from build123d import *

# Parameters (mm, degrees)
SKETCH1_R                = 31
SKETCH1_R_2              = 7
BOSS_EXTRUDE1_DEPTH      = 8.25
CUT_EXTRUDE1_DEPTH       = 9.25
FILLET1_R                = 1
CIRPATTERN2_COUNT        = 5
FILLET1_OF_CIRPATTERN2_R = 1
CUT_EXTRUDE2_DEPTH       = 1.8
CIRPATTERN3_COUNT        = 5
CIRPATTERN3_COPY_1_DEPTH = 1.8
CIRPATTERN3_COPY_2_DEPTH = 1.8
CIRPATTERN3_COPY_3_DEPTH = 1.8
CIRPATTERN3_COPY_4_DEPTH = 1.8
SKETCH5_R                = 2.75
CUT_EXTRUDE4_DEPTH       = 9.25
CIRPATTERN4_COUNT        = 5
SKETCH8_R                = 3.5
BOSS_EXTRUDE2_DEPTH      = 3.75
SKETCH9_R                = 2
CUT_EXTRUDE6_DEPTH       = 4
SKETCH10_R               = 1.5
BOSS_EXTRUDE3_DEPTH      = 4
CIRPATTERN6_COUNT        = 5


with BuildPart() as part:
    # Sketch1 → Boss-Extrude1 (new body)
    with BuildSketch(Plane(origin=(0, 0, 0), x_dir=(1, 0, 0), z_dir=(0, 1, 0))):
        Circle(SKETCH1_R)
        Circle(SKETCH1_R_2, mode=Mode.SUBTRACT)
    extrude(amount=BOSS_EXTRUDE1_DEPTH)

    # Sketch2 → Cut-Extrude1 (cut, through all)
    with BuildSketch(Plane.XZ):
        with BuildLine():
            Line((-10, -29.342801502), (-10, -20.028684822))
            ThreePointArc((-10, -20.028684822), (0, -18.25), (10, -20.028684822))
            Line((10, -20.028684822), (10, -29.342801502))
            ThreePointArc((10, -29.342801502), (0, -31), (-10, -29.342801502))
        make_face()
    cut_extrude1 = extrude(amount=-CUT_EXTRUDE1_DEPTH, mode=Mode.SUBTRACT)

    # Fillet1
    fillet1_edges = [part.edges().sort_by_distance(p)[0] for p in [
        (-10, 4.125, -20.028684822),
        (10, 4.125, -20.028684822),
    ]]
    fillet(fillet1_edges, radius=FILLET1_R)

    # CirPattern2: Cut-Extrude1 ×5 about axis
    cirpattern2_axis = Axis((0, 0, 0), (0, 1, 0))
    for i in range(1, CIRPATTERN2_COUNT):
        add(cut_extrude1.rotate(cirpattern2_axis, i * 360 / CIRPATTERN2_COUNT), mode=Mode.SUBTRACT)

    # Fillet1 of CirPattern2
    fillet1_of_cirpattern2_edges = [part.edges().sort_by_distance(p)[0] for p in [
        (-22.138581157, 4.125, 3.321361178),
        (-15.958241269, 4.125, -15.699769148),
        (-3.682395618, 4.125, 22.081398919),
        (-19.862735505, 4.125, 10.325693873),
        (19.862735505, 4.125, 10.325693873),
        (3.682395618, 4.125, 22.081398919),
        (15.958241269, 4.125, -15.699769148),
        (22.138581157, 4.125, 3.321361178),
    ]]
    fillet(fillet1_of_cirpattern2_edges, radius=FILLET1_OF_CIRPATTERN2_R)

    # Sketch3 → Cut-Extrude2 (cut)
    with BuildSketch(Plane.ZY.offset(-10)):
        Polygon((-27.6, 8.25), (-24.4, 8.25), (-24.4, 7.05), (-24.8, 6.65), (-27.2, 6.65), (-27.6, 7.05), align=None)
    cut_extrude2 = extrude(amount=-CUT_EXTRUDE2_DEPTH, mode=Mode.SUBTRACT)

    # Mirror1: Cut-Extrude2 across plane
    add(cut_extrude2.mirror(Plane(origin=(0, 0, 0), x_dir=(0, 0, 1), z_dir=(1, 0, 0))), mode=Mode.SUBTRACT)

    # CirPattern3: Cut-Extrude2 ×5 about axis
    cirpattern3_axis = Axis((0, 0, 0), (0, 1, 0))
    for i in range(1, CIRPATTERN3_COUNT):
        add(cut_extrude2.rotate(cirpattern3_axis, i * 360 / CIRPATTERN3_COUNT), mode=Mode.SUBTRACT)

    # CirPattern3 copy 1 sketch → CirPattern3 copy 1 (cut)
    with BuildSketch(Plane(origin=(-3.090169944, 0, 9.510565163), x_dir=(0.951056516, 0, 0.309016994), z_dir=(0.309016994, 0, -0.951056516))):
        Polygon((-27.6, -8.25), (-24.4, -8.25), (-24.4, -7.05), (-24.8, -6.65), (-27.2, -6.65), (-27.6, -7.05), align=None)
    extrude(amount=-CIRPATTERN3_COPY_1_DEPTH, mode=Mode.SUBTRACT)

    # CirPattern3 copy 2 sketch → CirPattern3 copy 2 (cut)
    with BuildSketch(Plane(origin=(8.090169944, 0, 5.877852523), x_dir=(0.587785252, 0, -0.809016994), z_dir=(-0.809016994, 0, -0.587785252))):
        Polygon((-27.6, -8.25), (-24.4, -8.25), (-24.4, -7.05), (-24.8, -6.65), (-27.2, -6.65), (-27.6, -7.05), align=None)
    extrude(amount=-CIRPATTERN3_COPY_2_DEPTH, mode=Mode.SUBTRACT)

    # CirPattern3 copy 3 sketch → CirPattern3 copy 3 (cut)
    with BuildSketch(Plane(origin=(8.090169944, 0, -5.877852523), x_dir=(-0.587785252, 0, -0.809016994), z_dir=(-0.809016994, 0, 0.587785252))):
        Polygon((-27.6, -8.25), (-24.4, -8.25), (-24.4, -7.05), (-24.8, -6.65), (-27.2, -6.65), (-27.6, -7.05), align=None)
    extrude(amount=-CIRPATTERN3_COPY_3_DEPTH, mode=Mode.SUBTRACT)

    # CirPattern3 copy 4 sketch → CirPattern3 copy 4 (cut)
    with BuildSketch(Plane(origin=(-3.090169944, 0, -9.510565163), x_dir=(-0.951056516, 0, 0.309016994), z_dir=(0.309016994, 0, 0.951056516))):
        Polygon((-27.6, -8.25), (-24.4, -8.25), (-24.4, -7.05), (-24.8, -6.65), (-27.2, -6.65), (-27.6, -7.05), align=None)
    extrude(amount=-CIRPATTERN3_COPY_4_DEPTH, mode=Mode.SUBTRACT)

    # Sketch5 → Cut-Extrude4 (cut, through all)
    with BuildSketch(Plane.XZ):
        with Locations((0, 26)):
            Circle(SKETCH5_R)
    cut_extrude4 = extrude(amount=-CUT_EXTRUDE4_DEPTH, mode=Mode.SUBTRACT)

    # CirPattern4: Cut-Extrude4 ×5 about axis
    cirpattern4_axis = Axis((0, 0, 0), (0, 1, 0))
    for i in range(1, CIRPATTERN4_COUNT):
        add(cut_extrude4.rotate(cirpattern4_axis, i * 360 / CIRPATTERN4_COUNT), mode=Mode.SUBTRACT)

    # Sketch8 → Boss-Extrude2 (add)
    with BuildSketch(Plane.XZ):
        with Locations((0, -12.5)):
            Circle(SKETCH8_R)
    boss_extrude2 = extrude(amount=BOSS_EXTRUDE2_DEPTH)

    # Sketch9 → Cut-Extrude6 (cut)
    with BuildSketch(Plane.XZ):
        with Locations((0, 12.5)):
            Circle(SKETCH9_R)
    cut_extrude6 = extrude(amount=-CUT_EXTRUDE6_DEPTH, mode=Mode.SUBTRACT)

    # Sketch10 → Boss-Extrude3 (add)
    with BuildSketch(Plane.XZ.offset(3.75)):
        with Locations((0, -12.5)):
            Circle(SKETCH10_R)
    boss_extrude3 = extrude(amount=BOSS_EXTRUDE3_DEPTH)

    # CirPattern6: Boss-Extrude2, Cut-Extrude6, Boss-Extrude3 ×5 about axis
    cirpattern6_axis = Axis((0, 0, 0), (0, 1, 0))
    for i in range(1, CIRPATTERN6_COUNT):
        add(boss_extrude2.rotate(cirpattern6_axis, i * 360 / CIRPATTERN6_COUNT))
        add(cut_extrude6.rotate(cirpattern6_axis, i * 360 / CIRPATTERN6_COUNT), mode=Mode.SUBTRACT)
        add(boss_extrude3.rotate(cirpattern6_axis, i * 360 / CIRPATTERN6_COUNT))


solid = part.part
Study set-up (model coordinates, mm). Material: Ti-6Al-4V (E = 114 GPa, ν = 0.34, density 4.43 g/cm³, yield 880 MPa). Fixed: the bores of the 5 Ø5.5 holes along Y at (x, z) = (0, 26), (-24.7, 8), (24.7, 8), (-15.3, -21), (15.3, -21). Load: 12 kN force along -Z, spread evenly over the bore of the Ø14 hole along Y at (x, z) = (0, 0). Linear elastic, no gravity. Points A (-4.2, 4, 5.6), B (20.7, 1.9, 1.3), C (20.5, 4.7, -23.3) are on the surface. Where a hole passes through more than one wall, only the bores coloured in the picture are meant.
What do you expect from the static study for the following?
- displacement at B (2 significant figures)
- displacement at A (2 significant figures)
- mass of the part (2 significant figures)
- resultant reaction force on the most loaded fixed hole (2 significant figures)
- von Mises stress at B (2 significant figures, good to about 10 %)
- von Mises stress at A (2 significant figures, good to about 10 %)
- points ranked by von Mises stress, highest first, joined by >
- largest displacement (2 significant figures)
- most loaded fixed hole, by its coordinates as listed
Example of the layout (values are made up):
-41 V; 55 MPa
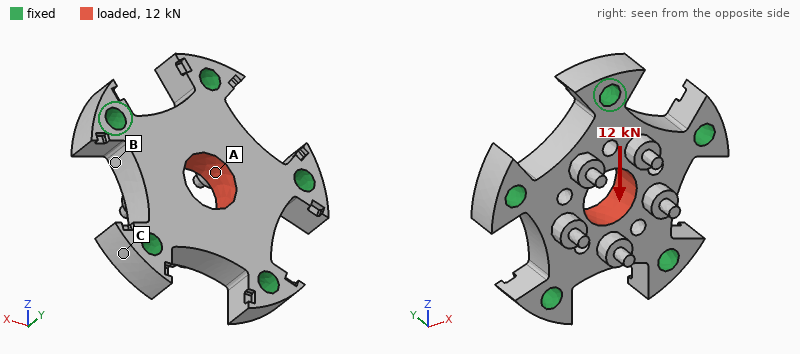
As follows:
1.6 µm; 7.4 µm; 60 g; 4.0 kN; 27 MPa; 42 MPa; A > B > C; 8.2 µm; (0, 26)
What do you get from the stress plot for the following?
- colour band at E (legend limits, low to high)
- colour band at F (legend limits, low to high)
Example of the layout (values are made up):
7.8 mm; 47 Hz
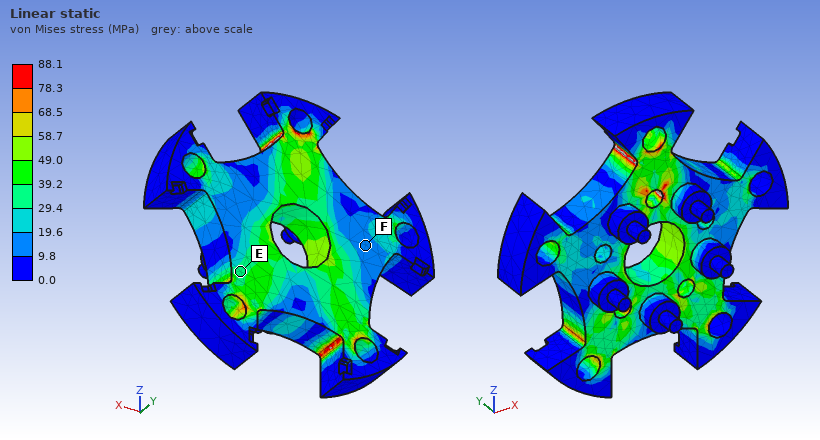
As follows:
29.4 to 39.2 MPa; 9.8 to 19.6 MPa
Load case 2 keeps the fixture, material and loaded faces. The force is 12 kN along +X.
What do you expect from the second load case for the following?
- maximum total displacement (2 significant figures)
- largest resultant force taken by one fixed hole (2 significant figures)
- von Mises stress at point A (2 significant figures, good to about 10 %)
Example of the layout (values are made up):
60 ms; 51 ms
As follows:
8.2 µm; 3.8 kN; 53 MPa
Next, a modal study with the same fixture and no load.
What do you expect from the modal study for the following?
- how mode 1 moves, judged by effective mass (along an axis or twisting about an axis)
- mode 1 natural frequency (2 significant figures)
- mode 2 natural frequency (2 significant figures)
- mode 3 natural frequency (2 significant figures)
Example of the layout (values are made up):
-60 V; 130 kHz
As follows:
along Y; 20 kHz; 31 kHz; 31 kHz
